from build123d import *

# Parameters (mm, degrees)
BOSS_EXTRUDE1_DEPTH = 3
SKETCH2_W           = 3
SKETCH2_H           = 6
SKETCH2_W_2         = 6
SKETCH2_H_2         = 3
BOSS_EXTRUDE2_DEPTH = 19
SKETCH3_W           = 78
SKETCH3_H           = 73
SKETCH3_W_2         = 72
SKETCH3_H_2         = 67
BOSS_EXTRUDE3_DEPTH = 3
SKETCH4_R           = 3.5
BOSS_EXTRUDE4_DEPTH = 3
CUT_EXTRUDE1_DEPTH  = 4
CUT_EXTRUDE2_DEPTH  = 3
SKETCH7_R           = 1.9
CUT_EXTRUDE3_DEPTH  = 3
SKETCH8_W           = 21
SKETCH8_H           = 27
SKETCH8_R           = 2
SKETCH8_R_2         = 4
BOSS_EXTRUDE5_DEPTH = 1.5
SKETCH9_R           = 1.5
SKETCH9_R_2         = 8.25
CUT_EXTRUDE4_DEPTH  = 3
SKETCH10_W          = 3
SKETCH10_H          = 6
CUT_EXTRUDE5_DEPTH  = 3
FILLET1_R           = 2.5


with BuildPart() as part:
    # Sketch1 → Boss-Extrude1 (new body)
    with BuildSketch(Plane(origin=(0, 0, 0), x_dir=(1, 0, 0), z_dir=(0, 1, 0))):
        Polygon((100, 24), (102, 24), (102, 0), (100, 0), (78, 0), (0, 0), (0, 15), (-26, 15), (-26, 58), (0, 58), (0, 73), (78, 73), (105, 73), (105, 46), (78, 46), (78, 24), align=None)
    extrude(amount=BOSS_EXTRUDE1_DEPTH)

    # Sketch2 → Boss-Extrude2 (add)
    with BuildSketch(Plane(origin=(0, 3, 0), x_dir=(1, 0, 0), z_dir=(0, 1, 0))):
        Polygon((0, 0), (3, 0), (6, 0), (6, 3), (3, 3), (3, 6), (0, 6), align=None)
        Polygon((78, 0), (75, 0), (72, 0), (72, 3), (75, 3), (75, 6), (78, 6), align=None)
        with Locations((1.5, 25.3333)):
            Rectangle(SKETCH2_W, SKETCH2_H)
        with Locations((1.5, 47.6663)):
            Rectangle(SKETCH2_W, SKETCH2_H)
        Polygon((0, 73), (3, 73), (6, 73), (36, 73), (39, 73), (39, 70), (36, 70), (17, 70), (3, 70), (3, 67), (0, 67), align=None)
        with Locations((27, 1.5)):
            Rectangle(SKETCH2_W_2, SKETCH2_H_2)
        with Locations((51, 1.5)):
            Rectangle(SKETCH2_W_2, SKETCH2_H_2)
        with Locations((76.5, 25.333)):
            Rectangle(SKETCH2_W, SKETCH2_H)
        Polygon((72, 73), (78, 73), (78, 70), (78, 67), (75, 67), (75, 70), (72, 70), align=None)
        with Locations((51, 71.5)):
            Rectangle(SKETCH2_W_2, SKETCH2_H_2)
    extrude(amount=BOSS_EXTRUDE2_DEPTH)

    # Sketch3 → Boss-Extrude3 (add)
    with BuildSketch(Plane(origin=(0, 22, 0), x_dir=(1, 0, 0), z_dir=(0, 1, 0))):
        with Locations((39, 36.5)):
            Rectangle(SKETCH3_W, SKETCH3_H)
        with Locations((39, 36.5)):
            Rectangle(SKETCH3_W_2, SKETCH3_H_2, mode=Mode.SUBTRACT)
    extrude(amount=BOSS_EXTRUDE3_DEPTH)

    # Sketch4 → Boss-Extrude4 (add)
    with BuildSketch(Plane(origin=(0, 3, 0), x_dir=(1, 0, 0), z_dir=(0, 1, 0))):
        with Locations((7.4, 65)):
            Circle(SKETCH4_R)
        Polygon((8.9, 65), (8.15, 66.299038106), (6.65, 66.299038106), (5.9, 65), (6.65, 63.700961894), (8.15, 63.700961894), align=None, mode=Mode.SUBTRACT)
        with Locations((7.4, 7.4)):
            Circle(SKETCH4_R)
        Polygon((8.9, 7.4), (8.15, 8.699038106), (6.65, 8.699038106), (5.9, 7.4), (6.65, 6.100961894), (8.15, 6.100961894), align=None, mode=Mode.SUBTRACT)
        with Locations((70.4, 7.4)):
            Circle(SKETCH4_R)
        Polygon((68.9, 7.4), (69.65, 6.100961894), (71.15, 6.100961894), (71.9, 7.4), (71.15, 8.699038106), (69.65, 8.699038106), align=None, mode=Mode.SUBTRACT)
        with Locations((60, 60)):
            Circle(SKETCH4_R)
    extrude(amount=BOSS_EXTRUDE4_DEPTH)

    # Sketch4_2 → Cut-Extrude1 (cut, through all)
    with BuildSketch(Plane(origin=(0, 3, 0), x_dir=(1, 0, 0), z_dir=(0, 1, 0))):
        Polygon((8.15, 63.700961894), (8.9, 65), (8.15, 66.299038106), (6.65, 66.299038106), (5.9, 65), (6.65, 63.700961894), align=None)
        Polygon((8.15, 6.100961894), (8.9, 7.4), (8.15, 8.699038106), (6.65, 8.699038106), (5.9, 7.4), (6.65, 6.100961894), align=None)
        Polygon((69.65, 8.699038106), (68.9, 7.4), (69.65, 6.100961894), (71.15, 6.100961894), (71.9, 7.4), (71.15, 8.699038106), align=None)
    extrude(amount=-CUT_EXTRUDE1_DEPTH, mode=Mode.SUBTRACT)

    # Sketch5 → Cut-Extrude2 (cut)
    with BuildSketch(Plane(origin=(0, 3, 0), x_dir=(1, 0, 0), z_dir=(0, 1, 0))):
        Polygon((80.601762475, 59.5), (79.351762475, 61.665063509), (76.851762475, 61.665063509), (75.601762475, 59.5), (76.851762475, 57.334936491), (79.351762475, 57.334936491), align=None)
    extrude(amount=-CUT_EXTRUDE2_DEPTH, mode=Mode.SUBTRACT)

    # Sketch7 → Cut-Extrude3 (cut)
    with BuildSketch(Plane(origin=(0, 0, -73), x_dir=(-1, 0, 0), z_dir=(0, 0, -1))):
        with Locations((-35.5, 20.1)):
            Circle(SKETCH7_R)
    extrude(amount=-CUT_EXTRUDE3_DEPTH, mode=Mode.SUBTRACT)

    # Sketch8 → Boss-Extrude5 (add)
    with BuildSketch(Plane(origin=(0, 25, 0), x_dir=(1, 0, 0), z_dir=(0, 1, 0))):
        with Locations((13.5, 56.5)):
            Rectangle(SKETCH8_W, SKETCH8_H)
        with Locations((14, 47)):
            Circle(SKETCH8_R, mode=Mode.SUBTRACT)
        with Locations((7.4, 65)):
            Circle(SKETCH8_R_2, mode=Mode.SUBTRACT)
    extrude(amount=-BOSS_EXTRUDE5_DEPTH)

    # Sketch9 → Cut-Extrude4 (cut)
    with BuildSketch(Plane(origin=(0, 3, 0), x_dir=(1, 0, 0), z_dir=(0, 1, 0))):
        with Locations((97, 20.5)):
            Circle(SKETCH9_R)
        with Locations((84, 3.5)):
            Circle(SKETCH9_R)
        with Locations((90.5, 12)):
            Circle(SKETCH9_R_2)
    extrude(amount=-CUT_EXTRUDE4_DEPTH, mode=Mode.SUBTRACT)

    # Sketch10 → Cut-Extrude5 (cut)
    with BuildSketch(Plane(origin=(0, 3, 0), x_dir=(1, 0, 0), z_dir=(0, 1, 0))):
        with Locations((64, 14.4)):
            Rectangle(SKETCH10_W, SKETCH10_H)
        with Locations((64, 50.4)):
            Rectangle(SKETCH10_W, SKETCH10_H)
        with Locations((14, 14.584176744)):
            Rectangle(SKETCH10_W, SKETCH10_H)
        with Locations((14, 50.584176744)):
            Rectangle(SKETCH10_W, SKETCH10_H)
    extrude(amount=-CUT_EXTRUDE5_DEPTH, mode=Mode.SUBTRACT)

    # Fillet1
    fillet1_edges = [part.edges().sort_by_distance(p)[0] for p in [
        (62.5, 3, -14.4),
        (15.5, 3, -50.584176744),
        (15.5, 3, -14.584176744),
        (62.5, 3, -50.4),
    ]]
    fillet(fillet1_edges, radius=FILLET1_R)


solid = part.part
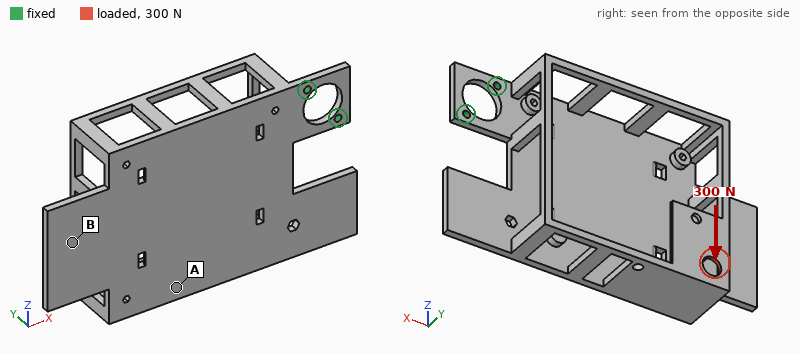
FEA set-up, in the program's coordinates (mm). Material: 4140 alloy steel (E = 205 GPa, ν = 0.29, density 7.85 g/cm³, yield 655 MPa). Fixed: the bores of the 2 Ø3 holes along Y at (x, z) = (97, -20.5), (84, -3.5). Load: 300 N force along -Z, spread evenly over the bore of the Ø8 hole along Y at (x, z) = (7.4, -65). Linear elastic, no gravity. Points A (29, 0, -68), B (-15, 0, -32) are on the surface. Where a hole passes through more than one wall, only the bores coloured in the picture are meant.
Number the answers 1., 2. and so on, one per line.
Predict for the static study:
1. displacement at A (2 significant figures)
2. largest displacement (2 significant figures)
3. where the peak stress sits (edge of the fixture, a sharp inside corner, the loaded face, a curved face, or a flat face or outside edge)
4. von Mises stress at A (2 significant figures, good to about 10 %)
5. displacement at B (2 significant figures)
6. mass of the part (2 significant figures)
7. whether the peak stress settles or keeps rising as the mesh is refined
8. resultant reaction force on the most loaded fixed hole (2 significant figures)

1. 0.65 mm
2. 0.93 mm
3. edge of the fixture
4. 34 MPa
5. 0.47 mm
6. 260 g
7. keeps rising
8. 1.2 kN
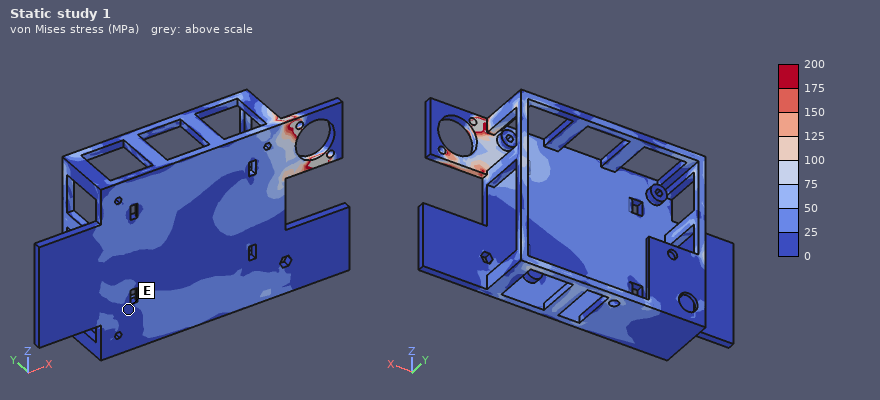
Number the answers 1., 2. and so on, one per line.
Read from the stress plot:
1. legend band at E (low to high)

1. 0 to 25 MPa
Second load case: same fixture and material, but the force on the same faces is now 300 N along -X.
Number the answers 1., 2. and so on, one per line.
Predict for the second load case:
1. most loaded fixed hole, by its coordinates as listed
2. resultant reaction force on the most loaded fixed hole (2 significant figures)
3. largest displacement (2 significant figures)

1. (97, -20.5)
2. 940 N
3. 1.5 mm
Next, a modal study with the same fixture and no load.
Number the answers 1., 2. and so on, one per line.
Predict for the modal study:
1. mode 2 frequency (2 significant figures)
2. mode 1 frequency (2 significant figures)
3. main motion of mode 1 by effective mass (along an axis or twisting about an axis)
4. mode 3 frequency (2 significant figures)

1. 380 Hz
2. 120 Hz
3. along Y
4. 740 Hz
